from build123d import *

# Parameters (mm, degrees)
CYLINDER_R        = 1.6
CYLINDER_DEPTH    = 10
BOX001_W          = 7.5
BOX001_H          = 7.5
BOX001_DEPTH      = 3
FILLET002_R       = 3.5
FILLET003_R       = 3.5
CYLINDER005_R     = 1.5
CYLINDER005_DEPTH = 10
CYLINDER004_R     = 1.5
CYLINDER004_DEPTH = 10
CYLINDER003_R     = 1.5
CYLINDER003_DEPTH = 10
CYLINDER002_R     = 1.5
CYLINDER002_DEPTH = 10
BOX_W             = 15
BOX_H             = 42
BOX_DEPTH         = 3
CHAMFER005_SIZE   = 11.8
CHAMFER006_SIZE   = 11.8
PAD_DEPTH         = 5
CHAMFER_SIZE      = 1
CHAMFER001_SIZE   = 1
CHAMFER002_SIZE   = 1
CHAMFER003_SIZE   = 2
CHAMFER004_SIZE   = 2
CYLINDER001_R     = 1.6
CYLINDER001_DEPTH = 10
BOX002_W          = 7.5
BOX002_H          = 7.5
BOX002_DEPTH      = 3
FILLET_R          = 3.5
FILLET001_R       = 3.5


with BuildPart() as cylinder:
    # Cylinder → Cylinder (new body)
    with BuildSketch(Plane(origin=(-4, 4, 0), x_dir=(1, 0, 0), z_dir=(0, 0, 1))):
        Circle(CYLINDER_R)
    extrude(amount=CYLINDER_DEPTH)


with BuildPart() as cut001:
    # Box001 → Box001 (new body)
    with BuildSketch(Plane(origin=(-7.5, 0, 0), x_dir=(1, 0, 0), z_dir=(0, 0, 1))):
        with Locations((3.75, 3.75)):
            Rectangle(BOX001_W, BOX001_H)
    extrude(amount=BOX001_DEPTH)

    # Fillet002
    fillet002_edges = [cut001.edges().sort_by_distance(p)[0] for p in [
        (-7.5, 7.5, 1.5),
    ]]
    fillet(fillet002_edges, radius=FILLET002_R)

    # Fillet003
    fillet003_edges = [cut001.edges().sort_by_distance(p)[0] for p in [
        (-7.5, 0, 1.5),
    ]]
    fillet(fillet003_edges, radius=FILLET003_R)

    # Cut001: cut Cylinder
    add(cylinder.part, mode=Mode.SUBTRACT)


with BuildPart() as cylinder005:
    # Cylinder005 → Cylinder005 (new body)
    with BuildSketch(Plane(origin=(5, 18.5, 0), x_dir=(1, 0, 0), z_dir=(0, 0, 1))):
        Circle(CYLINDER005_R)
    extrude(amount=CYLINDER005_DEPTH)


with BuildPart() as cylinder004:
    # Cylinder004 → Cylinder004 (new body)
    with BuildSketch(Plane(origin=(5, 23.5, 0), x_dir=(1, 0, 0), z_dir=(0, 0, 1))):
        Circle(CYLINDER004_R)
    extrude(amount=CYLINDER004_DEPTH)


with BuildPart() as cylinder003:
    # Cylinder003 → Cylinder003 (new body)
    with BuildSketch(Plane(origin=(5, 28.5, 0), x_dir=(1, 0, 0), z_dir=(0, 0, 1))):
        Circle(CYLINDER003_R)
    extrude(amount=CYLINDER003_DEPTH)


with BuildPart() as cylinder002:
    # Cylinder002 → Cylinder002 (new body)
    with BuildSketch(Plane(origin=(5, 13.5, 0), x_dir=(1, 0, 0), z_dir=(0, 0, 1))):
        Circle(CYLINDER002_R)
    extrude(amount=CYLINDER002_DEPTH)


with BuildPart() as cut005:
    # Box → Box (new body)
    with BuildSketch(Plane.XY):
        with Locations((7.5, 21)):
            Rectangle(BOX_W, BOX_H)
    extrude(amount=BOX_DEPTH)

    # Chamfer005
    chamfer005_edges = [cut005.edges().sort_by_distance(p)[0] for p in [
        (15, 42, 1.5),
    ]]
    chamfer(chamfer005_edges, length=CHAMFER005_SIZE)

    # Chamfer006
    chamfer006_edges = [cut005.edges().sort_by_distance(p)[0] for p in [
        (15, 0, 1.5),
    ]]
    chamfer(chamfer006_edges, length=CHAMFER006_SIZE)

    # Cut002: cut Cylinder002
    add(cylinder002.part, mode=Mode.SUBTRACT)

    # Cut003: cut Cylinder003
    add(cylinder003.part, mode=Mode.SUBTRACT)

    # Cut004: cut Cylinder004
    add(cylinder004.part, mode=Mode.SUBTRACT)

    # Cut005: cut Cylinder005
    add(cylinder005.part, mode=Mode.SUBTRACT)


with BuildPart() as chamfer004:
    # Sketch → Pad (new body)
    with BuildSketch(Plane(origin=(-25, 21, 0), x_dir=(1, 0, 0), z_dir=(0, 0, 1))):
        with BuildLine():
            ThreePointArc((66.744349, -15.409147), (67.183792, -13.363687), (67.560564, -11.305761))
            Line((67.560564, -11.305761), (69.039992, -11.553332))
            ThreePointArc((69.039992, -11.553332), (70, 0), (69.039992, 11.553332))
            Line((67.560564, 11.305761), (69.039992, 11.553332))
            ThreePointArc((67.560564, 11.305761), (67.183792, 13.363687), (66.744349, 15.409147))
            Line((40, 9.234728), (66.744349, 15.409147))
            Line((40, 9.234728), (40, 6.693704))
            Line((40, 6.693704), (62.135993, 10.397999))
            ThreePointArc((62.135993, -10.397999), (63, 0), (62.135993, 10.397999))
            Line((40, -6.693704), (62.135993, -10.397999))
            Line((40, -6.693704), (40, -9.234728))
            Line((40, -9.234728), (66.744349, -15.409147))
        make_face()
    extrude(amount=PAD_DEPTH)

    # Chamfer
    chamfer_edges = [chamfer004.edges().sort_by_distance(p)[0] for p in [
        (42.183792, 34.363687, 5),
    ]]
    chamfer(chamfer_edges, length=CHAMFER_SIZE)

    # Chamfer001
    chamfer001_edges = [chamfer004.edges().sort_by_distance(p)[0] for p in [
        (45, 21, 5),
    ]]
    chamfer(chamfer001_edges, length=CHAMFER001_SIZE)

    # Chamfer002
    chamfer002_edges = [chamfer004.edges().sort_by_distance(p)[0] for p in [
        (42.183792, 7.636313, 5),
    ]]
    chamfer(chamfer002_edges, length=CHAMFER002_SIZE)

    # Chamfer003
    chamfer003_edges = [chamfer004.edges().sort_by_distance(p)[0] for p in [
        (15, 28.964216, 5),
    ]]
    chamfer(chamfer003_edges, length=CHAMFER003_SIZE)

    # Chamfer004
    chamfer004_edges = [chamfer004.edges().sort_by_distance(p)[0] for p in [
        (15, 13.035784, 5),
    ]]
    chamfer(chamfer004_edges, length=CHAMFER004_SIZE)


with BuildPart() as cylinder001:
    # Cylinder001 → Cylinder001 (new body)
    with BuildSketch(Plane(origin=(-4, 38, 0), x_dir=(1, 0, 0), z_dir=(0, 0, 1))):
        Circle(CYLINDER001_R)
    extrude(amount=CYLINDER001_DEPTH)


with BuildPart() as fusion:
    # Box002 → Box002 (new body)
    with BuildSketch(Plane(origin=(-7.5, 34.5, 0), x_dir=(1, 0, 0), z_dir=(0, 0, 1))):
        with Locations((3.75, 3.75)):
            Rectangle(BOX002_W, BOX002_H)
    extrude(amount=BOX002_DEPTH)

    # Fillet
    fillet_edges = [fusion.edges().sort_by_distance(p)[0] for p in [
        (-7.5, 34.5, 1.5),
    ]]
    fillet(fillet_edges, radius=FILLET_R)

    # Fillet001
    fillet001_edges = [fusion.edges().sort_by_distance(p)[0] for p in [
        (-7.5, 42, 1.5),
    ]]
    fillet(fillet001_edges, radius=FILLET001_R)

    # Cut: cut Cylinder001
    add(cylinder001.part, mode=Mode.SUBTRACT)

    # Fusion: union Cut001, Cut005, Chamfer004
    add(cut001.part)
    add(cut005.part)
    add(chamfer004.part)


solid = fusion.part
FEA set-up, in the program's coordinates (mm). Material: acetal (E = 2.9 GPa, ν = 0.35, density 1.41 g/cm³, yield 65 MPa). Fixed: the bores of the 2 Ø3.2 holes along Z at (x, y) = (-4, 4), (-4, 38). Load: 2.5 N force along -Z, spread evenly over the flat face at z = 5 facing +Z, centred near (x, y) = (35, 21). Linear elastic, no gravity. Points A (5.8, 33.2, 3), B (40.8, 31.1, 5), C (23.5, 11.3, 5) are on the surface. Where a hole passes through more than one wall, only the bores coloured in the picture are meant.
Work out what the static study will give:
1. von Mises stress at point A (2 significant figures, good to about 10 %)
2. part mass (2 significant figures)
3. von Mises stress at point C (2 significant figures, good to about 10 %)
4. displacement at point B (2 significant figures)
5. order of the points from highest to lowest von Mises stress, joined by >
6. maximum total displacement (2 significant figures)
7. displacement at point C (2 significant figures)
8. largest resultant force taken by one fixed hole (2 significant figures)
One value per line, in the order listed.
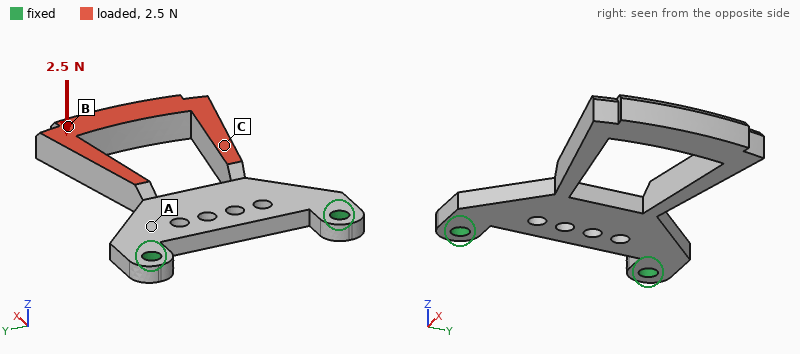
2.5 MPa
4.7 g
1.2 MPa
0.63 mm
A > C > B
0.71 mm
0.30 mm
1.3 N
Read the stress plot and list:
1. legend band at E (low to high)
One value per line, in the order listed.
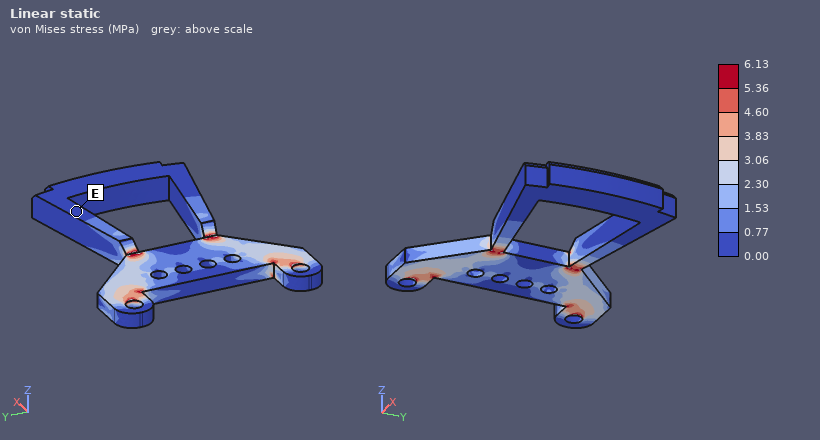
0.00 to 0.77 MPa
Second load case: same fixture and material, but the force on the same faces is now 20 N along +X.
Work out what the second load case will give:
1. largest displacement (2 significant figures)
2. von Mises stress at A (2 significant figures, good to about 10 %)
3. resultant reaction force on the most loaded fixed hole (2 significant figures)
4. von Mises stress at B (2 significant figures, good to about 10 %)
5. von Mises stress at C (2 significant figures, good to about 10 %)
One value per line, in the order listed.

0.74 mm
3.0 MPa
11 N
0.76 MPa
2.4 MPa
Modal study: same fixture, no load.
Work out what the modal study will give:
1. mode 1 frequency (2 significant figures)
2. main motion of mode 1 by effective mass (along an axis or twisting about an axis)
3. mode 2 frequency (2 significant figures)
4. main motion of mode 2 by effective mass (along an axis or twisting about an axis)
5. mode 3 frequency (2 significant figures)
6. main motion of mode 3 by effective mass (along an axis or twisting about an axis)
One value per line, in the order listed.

220 Hz
along Z
590 Hz
along Y
780 Hz
twisting about X
